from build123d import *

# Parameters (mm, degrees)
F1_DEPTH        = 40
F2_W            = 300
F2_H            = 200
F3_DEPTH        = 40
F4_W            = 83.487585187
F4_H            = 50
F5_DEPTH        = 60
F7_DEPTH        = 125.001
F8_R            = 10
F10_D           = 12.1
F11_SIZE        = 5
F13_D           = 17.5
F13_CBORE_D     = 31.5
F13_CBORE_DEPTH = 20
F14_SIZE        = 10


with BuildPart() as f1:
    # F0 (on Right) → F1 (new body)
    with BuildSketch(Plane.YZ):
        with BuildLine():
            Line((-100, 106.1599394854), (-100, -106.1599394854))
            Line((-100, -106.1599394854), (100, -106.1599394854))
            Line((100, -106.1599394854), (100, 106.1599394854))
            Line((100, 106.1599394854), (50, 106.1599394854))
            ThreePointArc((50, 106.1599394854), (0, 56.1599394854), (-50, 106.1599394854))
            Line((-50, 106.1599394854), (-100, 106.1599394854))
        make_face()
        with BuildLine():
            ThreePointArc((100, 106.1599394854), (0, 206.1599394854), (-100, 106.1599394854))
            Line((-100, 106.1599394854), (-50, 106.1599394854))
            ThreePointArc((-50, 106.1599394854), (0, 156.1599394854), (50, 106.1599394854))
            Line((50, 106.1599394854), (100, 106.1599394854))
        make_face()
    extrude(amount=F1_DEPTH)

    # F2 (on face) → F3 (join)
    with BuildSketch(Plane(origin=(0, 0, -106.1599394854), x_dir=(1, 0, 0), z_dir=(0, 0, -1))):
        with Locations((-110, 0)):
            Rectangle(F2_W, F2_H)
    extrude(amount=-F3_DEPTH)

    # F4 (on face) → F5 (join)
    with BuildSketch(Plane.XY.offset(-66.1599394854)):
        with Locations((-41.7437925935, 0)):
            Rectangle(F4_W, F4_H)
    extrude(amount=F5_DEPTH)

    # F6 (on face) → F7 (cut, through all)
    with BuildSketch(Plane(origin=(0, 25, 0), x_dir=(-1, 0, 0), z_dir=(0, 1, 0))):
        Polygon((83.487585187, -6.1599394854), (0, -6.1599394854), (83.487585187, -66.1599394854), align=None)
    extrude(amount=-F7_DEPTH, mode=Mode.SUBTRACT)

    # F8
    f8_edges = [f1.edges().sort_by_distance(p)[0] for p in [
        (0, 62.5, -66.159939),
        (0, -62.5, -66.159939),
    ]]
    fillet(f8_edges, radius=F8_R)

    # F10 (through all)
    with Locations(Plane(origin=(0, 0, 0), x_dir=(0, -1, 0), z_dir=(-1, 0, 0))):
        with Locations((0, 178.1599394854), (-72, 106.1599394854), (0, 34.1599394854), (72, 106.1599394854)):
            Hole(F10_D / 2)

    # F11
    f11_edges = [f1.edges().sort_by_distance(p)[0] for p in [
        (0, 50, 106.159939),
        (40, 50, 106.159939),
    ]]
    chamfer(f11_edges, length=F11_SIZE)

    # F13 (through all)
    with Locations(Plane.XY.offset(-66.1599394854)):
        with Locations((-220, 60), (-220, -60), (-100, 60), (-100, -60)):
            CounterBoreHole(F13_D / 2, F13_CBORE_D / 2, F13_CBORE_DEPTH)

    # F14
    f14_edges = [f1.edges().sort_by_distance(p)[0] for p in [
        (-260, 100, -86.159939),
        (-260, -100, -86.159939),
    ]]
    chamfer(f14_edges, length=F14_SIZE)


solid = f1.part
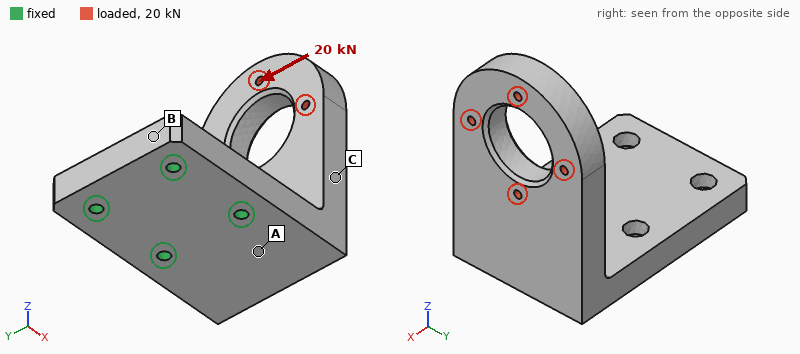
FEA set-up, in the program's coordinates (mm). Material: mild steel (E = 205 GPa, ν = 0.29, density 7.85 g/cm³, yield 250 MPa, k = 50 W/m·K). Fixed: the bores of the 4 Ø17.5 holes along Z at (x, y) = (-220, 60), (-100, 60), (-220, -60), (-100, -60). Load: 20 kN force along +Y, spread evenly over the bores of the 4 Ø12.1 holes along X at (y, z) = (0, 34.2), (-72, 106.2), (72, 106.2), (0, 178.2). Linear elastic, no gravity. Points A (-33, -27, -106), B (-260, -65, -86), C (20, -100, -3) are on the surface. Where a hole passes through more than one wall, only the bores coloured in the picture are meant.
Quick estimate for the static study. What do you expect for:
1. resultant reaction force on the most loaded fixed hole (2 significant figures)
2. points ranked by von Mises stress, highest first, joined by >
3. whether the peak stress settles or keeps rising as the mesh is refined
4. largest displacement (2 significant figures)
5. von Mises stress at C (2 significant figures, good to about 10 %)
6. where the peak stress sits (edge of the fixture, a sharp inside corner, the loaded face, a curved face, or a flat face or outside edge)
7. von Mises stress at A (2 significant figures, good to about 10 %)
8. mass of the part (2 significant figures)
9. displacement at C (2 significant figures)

40 kN
A > C > B
keeps rising
0.24 mm
11 MPa
edge of the fixture
31 MPa
32 kg
0.097 mm
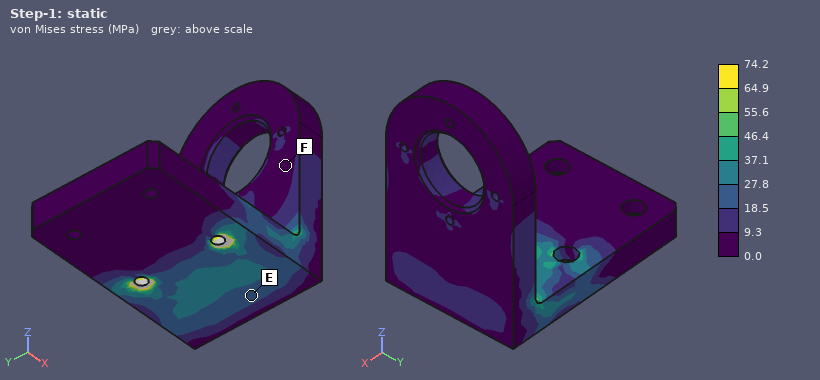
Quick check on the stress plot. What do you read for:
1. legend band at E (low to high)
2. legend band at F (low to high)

18.5 to 27.8 MPa
0.0 to 9.3 MPa
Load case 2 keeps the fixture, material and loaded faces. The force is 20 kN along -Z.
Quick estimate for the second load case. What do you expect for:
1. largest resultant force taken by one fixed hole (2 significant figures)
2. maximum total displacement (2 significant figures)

21 kN
0.25 mm
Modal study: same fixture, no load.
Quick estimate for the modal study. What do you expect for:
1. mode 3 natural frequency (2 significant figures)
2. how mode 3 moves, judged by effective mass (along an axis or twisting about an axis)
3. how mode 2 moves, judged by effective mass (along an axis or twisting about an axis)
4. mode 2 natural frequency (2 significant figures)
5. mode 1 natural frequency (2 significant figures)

950 Hz
along Z
along Y
570 Hz
320 Hz
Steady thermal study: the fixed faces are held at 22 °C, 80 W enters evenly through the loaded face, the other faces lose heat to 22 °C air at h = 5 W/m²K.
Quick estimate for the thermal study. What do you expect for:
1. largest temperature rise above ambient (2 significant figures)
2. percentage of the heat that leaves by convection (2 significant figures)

55 K
33 %
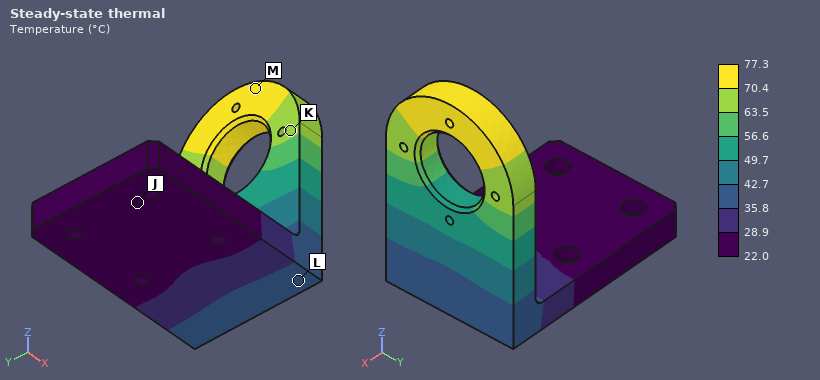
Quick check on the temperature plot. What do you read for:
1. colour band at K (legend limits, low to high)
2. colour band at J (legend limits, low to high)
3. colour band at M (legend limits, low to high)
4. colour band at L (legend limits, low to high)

63.5 to 70.4 °C
22.0 to 28.9 °C
70.4 to 77.3 °C
35.8 to 42.7 °C
